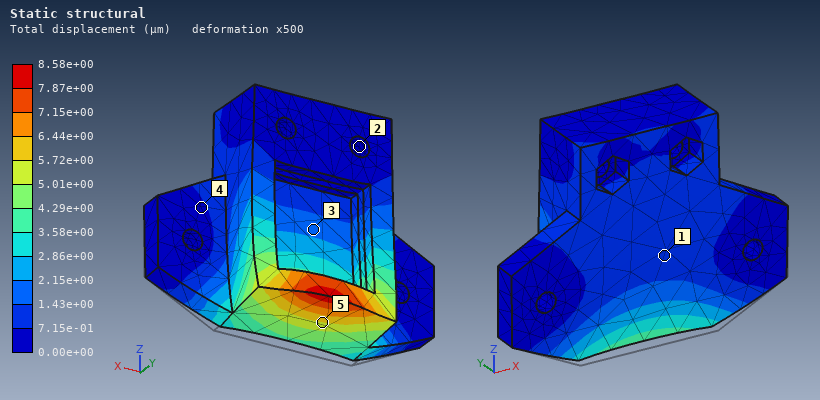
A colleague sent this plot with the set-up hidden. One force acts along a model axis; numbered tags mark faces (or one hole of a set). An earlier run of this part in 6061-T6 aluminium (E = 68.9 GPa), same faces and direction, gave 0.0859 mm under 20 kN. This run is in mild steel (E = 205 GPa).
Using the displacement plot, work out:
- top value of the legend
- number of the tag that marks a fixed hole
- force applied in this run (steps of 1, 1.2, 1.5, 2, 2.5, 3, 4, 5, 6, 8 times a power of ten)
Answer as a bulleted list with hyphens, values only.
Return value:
- 8.58e+00 µm
- 2
- 6 kN
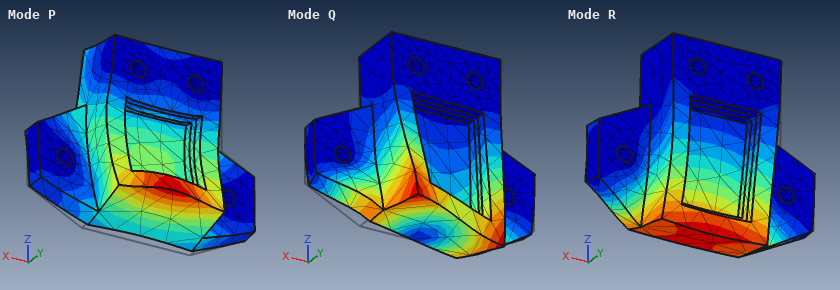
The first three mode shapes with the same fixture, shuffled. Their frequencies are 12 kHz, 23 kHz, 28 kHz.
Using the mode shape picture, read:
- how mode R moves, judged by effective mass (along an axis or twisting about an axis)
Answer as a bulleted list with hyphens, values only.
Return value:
- along Y
